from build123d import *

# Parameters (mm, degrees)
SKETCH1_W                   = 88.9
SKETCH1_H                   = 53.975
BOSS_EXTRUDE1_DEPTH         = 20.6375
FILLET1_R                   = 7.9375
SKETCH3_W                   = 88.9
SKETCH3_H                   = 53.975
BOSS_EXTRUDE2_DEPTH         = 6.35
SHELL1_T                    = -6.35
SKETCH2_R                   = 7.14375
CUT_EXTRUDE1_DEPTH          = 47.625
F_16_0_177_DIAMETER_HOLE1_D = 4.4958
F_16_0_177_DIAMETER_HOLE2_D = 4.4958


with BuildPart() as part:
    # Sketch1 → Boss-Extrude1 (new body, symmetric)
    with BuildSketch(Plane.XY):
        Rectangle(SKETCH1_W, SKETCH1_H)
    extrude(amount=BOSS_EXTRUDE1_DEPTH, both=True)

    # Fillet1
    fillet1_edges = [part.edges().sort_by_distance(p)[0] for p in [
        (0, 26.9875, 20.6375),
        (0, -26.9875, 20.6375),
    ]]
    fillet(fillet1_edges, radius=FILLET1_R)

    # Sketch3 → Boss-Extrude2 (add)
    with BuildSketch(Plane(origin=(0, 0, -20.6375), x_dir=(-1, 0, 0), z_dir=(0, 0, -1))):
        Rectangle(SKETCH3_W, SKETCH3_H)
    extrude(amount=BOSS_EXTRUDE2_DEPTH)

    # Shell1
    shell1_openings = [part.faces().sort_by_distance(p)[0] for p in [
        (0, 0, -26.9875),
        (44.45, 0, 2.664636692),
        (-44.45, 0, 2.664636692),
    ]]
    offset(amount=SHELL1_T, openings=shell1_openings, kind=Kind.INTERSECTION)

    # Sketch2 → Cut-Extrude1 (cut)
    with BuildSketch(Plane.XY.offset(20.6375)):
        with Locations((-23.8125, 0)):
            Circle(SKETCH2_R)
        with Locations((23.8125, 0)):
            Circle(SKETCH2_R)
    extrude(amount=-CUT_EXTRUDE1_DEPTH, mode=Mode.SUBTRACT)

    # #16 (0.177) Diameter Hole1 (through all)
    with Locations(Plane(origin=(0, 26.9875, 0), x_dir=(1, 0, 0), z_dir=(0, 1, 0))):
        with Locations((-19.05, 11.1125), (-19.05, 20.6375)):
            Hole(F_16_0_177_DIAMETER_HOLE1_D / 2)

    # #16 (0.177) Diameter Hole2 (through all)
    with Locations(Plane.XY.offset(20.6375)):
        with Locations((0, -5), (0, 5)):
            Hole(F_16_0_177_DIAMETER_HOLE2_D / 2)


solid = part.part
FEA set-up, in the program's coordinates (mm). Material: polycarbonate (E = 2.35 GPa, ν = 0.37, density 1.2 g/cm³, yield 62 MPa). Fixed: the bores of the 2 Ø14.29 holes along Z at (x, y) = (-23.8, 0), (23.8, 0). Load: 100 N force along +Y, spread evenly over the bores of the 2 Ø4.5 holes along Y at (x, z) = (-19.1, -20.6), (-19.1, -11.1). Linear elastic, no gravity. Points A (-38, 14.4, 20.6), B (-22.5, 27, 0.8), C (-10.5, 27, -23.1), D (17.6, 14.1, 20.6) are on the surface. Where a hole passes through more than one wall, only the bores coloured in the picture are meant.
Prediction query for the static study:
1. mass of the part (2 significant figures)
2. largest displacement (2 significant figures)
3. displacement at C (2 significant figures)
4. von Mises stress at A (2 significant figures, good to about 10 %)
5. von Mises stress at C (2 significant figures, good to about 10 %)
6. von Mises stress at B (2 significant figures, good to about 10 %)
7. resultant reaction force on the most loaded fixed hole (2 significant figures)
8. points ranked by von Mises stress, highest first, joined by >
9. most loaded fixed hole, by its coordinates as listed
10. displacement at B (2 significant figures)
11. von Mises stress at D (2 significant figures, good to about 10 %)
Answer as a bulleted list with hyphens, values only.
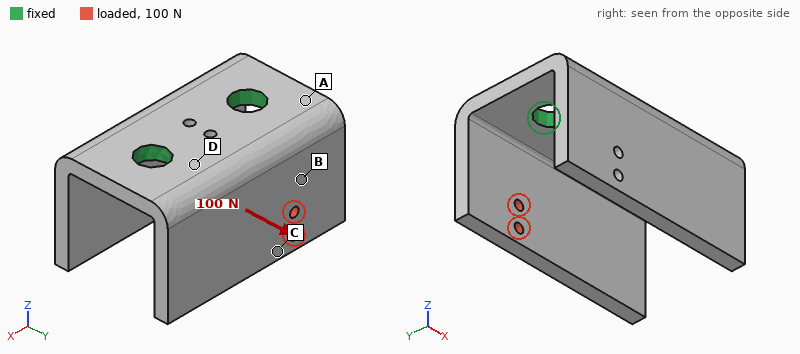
- 87 g
- 1.2 mm
- 0.98 mm
- 5.9 MPa
- 2.2 MPa
- 3.2 MPa
- 86 N
- A > D > B > C
- (-23.8, 0)
- 0.43 mm
- 4.4 MPa
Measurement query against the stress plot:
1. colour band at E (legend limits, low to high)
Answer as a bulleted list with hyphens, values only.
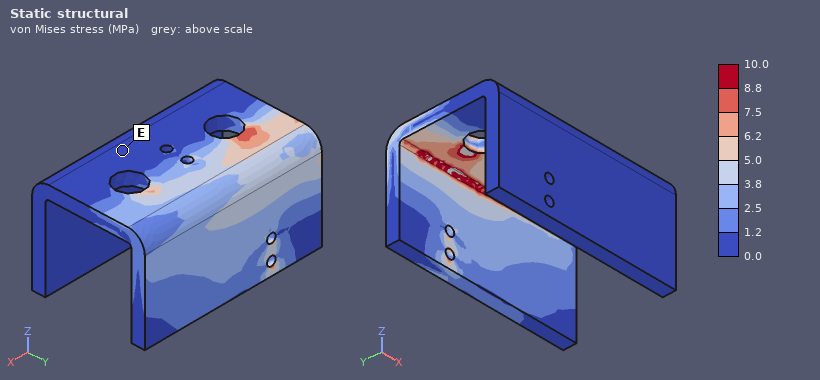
- 0.0 to 1.2 MPa
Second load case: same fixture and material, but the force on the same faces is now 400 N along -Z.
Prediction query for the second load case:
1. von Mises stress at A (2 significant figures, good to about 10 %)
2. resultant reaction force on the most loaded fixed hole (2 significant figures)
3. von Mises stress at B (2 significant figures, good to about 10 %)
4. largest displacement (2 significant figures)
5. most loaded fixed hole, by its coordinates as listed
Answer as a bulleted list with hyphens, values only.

- 6.9 MPa
- 340 N
- 1.9 MPa
- 1.1 mm
- (-23.8, 0)
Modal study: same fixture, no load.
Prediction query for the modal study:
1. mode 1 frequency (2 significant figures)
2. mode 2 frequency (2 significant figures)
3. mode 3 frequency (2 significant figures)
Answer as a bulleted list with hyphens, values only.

- 450 Hz
- 450 Hz
- 760 Hz
